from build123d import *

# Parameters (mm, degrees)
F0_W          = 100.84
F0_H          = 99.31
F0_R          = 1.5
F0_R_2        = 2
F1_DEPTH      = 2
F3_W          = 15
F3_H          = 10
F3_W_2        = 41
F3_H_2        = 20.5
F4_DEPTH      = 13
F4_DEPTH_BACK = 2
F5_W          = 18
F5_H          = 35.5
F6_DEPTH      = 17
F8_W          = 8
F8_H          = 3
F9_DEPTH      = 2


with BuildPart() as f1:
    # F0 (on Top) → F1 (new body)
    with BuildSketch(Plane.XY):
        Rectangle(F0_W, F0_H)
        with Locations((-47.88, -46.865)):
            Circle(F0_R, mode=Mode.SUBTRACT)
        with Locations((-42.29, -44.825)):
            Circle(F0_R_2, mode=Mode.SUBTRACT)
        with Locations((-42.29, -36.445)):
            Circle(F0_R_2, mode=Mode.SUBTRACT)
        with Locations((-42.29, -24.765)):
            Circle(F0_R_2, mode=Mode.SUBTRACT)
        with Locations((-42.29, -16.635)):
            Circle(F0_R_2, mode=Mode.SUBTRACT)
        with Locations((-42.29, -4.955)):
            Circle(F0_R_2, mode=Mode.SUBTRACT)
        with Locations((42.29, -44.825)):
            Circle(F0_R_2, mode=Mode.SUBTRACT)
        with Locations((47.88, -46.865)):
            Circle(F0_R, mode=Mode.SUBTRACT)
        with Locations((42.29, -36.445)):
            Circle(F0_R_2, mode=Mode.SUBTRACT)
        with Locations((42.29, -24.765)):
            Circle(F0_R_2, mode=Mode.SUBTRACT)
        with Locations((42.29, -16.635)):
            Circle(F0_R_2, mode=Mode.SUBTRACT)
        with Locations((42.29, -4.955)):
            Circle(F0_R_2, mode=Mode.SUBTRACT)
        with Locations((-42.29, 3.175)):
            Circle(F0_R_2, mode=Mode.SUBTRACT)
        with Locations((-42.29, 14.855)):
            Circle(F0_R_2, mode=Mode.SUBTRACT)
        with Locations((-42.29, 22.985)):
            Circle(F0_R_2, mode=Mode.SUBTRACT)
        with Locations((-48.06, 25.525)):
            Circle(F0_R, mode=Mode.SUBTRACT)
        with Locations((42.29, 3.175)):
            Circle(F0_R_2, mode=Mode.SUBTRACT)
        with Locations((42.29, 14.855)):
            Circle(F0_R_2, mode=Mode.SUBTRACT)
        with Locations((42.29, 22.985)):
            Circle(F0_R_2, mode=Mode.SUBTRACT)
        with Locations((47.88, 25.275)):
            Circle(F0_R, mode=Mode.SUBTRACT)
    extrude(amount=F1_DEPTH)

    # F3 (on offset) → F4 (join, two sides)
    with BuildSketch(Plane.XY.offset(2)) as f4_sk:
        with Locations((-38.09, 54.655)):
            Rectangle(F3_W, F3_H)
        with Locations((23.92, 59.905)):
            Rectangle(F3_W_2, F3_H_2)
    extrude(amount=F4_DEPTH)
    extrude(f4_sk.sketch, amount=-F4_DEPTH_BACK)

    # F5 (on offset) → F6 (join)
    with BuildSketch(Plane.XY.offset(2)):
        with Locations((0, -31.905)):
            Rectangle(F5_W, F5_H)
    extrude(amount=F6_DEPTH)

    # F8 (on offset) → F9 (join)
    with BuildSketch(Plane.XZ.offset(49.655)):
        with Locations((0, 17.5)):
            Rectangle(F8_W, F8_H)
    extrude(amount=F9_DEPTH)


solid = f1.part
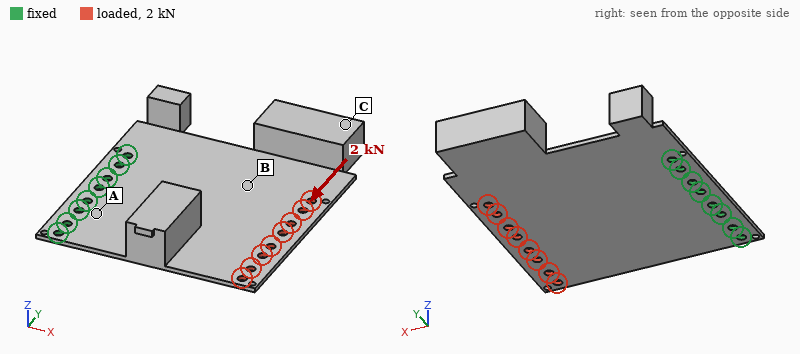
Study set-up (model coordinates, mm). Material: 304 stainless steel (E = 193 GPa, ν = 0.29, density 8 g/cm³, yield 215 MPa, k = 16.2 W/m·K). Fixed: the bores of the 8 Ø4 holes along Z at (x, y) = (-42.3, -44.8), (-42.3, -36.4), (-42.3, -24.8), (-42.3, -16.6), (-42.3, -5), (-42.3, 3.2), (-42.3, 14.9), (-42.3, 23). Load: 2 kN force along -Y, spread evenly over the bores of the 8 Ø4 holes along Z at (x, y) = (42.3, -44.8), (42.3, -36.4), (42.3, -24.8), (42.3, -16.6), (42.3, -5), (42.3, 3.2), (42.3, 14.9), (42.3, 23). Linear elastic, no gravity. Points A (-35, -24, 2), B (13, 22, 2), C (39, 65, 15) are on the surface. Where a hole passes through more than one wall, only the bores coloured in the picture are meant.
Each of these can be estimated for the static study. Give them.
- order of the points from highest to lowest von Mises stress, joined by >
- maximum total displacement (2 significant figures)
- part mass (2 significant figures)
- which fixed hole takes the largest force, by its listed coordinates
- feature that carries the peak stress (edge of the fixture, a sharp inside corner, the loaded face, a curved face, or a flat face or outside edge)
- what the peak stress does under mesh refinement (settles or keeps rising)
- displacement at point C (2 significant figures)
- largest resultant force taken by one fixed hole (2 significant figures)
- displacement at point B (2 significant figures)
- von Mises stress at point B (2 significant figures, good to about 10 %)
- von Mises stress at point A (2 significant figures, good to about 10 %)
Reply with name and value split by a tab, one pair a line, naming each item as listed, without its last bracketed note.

order of the points from highest to lowest von Mises stress, joined by >	A > B > C
maximum total displacement	46 µm
part mass	360 g
which fixed hole takes the largest force, by its listed coordinates	(-42.3, 23)
feature that carries the peak stress	edge of the fixture
what the peak stress does under mesh refinement	keeps rising
displacement at point C	43 µm
largest resultant force taken by one fixed hole	2.0 kN
displacement at point B	24 µm
von Mises stress at point B	19 MPa
von Mises stress at point A	33 MPa
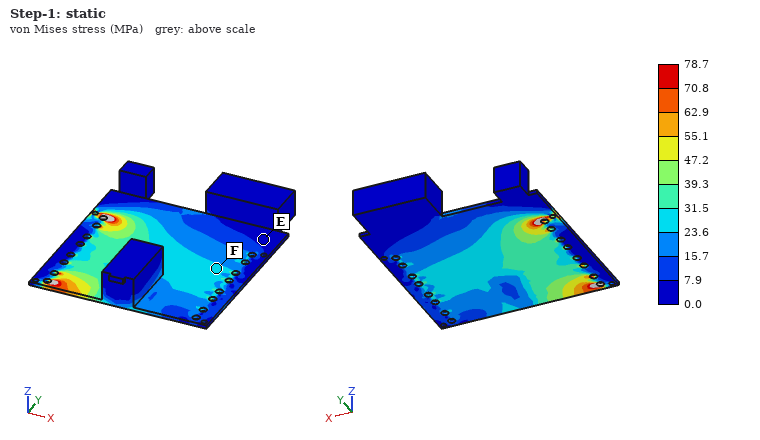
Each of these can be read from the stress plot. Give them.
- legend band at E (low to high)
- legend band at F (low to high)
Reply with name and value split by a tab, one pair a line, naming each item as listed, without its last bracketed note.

legend band at E	0.0 to 7.9 MPa
legend band at F	23.6 to 31.5 MPa
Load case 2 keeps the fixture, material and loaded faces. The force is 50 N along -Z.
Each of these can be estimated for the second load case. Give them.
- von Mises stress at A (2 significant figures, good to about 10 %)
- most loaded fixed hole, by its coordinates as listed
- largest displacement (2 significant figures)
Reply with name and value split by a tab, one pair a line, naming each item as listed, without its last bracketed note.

von Mises stress at A	58 MPa
most loaded fixed hole, by its coordinates as listed	(-42.3, 14.9)
largest displacement	0.78 mm
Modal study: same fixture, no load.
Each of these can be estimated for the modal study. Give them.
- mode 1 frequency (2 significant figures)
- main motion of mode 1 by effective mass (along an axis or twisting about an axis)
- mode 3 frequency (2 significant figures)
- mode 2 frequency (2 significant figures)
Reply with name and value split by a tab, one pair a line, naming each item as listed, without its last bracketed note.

mode 1 frequency	110 Hz
main motion of mode 1 by effective mass	along Z
mode 3 frequency	580 Hz
mode 2 frequency	230 Hz
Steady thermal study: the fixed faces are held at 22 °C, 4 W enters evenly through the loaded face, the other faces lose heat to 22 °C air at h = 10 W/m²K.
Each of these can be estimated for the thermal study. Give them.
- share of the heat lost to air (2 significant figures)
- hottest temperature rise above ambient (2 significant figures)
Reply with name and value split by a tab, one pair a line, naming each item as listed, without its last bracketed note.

share of the heat lost to air	83 %
hottest temperature rise above ambient	49 K
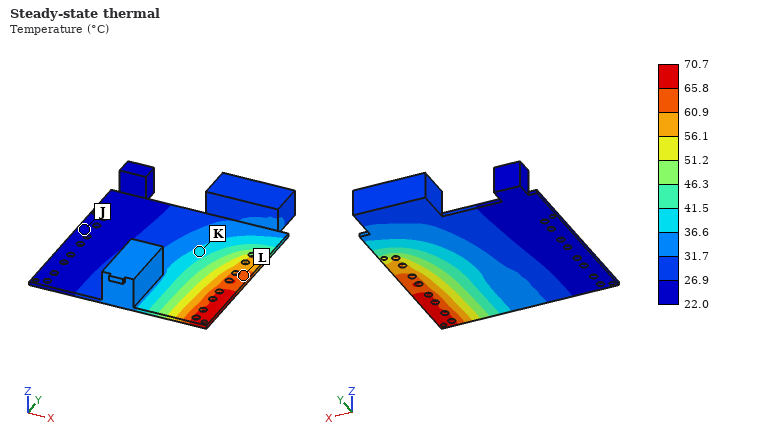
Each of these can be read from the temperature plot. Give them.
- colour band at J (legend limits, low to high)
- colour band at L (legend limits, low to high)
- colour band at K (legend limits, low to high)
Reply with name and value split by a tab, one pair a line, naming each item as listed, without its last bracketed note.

colour band at J	22.0 to 26.9 °C
colour band at L	60.9 to 65.8 °C
colour band at K	36.6 to 41.5 °C
